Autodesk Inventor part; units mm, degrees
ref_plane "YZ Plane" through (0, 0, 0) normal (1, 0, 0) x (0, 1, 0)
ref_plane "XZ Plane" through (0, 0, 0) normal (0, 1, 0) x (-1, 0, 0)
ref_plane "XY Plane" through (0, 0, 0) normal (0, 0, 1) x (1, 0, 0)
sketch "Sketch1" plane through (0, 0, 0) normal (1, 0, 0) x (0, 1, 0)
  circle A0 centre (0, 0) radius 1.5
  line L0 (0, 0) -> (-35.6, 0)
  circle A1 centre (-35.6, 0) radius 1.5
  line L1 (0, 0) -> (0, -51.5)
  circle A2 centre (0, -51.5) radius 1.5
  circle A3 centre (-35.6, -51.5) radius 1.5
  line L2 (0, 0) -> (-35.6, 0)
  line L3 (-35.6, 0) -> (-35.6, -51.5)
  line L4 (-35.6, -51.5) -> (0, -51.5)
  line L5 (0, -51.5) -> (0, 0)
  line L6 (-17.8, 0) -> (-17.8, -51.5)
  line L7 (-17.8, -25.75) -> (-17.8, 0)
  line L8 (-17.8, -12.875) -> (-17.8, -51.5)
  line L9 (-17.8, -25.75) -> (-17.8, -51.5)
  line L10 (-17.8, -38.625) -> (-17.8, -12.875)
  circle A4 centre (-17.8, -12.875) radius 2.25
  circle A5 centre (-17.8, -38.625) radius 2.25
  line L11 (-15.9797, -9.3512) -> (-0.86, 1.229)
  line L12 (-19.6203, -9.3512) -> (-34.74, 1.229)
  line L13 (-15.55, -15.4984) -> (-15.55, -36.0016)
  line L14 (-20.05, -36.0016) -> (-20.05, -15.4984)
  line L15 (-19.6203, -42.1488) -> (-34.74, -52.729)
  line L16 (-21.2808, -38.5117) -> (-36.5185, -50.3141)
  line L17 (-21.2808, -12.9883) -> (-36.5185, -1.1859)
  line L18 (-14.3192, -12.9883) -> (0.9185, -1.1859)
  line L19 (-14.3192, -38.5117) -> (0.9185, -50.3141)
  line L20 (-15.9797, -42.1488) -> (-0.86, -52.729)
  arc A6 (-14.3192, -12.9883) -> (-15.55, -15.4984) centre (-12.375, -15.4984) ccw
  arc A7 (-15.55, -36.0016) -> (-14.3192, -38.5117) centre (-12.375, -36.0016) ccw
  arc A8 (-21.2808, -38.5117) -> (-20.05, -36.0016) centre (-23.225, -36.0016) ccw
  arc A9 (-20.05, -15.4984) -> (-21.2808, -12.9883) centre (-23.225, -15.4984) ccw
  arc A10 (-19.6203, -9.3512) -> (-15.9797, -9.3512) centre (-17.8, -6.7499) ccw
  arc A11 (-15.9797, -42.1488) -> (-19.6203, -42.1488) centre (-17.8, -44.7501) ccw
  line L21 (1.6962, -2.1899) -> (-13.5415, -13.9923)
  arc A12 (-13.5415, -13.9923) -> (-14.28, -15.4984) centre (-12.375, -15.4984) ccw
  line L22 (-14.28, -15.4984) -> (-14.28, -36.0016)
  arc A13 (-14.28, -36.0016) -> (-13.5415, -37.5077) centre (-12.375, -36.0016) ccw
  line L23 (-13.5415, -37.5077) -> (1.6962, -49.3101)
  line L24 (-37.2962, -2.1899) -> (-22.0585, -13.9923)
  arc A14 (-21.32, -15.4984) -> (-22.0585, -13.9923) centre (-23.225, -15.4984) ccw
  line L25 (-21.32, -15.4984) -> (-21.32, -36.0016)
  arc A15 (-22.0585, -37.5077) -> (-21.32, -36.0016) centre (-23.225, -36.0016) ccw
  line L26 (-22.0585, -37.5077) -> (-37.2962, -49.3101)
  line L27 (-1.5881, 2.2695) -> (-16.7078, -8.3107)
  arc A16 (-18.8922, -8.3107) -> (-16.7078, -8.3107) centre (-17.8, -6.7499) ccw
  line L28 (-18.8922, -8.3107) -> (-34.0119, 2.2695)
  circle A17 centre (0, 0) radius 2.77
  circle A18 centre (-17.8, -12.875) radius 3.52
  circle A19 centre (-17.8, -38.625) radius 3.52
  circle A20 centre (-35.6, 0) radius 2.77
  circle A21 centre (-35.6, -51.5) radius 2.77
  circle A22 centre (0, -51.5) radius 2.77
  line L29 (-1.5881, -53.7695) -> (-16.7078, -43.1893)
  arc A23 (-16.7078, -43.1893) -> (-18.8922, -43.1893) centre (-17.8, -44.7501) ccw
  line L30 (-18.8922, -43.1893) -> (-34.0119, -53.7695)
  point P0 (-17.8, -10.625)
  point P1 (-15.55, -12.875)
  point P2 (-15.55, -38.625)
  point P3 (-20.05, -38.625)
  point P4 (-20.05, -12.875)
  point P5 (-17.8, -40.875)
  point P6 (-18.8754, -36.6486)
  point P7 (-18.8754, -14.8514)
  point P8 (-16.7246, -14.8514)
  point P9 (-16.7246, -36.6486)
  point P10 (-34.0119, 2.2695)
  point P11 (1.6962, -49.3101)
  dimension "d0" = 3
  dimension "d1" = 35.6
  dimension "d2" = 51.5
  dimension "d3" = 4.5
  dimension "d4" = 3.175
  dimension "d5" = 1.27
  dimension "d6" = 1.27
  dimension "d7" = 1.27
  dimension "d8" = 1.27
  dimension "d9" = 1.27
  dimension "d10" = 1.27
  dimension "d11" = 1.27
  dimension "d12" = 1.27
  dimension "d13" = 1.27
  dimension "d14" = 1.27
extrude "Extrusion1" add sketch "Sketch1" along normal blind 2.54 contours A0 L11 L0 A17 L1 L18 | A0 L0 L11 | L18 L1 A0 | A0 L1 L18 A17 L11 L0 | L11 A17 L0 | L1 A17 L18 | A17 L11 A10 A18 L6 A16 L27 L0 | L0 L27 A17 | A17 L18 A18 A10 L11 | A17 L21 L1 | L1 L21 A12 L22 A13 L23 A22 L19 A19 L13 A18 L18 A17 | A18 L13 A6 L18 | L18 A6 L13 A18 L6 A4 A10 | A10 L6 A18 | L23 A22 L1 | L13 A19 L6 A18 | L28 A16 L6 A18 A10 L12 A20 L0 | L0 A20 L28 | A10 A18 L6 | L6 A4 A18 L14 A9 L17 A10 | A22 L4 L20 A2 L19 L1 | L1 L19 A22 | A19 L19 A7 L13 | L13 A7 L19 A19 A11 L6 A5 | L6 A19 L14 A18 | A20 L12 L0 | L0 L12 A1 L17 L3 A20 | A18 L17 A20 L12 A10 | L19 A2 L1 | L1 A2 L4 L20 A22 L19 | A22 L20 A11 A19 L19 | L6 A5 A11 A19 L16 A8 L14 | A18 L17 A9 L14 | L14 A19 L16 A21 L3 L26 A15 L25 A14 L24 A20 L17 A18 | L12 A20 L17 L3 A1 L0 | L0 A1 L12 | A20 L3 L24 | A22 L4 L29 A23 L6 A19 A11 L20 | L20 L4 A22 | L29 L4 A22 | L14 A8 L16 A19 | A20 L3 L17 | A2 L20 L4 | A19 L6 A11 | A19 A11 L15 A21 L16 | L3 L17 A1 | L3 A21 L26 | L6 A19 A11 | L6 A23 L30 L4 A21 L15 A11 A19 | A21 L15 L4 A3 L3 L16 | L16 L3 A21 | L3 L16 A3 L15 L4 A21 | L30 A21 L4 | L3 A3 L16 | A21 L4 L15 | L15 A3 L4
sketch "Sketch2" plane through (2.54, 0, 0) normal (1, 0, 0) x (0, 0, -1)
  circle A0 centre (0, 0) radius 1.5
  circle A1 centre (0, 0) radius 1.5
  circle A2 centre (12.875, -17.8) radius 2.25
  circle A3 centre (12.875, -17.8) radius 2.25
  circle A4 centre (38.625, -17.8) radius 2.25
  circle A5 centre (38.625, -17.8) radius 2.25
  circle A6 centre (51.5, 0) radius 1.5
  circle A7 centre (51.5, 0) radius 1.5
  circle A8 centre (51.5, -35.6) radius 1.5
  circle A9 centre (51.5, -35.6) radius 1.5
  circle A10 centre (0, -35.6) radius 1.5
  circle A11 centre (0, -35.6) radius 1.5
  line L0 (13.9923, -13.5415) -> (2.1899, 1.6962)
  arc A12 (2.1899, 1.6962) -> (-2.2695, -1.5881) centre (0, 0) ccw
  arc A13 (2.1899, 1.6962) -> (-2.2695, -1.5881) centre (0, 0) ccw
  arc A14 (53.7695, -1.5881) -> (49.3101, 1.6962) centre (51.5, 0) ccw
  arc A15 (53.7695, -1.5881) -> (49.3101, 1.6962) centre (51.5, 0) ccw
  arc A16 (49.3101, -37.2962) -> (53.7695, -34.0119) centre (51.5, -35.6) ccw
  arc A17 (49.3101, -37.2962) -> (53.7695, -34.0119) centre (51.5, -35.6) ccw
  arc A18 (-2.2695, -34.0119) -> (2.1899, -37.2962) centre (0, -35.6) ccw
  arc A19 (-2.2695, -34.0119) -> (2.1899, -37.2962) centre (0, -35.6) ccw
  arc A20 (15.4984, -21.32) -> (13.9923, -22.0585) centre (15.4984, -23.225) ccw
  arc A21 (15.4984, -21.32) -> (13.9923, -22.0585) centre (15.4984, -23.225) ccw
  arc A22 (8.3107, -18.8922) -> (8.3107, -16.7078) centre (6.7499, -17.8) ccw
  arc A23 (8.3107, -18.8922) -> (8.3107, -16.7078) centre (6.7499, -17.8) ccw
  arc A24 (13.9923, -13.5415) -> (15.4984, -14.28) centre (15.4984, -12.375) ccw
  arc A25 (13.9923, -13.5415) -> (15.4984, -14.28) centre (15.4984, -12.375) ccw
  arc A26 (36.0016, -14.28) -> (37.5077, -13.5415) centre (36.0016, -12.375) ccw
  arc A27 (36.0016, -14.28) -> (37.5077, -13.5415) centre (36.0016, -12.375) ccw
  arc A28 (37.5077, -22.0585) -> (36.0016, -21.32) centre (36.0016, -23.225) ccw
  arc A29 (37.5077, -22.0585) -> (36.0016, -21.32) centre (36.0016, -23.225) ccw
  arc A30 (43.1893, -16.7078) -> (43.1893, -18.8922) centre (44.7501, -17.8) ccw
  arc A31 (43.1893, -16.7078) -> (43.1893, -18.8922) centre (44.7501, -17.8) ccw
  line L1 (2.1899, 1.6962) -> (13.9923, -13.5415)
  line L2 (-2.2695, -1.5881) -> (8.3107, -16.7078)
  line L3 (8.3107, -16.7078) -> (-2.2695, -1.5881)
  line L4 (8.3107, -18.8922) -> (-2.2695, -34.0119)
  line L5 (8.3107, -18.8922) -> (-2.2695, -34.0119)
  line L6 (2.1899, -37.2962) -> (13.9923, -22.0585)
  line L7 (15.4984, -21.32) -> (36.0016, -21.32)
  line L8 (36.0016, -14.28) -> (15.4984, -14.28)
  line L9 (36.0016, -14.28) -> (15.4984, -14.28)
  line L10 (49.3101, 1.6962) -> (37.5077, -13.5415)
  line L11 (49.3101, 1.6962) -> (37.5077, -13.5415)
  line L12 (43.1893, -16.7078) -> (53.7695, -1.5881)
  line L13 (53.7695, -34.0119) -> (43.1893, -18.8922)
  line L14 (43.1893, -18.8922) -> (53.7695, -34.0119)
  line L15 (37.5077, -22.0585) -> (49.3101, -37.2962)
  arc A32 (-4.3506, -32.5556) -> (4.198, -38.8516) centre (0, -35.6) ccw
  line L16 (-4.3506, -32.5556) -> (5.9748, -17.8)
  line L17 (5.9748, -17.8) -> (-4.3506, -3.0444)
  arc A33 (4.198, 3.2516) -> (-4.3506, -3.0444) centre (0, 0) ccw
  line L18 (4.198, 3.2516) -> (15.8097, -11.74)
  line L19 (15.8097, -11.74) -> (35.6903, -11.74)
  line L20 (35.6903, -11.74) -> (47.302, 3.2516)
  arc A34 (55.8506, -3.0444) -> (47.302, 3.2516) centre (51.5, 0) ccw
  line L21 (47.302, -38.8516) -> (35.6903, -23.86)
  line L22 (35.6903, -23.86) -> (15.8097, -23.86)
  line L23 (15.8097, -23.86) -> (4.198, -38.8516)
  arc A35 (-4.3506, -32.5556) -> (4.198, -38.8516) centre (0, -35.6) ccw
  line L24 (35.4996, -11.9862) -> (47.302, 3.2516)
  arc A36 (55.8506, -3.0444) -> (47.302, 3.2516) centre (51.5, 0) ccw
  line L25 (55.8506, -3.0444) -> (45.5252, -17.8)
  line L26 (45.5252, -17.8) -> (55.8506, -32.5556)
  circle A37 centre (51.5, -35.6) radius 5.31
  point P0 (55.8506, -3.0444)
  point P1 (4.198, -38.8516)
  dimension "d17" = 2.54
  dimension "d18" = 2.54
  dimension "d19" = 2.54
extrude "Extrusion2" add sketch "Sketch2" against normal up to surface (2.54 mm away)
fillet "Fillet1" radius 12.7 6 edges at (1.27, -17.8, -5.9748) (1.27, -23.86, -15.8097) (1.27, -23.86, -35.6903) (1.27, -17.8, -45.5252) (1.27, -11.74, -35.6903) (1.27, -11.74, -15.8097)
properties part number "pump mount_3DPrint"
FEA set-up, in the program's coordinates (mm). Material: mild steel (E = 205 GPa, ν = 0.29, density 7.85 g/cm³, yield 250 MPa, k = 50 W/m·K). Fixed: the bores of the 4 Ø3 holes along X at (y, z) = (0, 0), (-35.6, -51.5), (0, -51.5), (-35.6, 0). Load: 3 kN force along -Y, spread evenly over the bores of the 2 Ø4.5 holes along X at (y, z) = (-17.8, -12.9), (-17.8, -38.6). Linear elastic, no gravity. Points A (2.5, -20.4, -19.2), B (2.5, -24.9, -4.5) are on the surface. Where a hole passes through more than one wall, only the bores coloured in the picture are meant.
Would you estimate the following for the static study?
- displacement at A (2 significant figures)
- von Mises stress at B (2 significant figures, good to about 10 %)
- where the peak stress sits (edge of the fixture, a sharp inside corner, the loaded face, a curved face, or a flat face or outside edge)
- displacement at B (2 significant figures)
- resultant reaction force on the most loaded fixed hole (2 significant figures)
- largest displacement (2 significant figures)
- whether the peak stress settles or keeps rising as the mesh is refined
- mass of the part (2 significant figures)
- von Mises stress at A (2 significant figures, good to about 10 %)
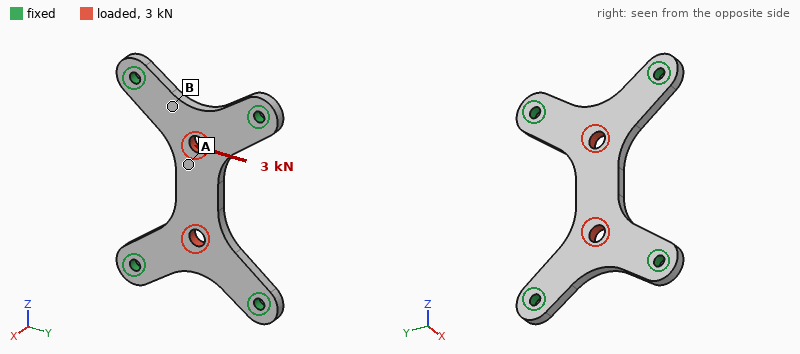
5.4 µm
26 MPa
edge of the fixture
2.0 µm
920 N
6.0 µm
keeps rising
27 g
11 MPa
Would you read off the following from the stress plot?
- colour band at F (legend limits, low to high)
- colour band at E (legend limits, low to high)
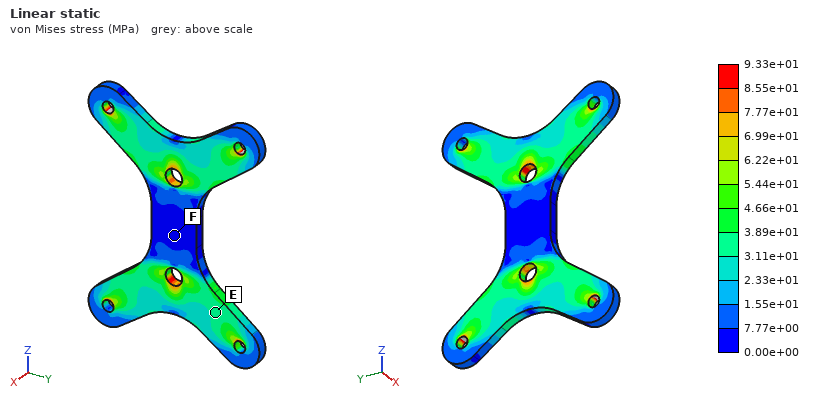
0.00e+00 to 7.77e+00 MPa
3.11e+01 to 3.89e+01 MPa
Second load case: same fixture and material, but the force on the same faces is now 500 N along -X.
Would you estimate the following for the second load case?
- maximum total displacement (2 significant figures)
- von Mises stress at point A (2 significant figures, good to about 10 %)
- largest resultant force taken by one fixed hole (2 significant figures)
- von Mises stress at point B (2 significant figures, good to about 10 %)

60 µm
54 MPa
130 N
40 MPa
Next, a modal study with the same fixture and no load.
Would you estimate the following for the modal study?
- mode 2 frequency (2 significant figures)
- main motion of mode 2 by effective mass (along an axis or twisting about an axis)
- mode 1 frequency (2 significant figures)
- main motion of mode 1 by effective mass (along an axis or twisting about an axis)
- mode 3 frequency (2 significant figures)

9100 Hz
twisting about Y
4500 Hz
along X
14 kHz
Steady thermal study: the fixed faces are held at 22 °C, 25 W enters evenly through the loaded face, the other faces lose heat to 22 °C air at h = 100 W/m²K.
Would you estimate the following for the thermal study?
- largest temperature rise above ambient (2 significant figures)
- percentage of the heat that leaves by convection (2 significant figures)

72 K
40 %
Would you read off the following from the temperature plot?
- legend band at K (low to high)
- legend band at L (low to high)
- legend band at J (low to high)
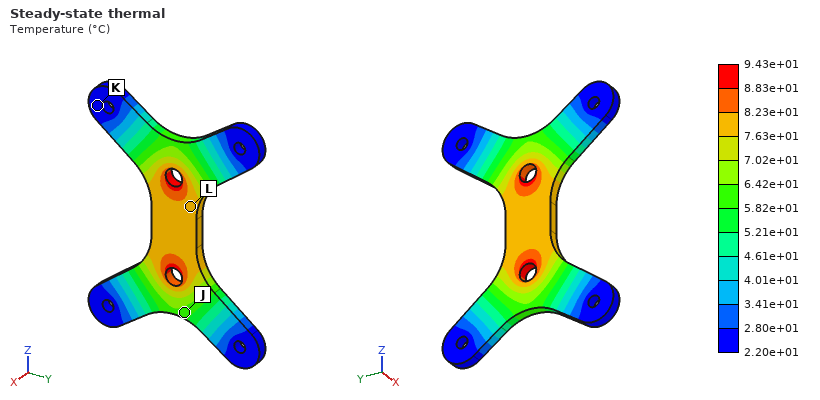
2.20e+01 to 2.80e+01 °C
7.63e+01 to 8.23e+01 °C
5.82e+01 to 6.42e+01 °C
